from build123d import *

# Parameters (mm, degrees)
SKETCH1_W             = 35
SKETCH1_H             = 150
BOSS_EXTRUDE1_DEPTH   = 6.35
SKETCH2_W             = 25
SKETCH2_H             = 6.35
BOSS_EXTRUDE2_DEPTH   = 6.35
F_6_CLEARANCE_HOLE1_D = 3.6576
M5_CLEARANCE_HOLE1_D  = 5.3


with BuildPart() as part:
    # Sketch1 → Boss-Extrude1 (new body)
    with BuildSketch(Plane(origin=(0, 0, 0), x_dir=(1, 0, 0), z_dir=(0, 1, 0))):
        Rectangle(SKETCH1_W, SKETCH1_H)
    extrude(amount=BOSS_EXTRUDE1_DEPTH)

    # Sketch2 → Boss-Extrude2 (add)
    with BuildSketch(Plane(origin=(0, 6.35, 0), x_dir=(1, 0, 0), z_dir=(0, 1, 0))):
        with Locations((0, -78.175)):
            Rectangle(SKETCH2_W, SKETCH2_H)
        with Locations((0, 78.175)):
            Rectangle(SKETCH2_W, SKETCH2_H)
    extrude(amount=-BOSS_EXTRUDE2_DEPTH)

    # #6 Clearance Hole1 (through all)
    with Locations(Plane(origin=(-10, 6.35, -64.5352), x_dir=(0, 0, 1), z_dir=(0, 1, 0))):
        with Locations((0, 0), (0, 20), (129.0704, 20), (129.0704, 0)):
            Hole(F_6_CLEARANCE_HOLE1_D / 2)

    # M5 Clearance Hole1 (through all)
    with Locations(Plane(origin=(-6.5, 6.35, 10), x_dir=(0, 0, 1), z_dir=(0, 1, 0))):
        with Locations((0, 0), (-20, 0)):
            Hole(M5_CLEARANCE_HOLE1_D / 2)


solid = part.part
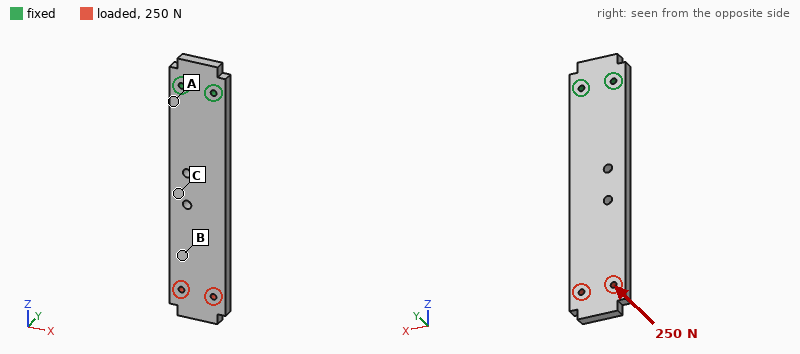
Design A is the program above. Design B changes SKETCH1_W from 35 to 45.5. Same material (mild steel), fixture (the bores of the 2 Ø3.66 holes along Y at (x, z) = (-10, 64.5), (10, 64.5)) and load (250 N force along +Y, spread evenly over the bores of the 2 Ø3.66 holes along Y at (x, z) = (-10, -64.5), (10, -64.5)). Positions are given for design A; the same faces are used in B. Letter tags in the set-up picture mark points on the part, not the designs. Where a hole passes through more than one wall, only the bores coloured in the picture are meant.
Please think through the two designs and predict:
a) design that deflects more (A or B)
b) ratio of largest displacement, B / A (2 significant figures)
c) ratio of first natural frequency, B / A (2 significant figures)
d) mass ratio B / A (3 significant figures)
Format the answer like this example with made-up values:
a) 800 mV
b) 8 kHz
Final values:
a) A
b) 0.78
c) 1.0
d) 1.29
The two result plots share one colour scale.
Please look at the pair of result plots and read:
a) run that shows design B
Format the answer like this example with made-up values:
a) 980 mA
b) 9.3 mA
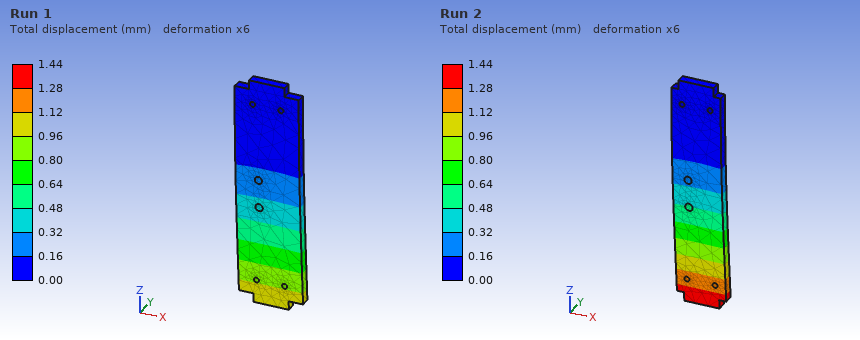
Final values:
a) Run 1
